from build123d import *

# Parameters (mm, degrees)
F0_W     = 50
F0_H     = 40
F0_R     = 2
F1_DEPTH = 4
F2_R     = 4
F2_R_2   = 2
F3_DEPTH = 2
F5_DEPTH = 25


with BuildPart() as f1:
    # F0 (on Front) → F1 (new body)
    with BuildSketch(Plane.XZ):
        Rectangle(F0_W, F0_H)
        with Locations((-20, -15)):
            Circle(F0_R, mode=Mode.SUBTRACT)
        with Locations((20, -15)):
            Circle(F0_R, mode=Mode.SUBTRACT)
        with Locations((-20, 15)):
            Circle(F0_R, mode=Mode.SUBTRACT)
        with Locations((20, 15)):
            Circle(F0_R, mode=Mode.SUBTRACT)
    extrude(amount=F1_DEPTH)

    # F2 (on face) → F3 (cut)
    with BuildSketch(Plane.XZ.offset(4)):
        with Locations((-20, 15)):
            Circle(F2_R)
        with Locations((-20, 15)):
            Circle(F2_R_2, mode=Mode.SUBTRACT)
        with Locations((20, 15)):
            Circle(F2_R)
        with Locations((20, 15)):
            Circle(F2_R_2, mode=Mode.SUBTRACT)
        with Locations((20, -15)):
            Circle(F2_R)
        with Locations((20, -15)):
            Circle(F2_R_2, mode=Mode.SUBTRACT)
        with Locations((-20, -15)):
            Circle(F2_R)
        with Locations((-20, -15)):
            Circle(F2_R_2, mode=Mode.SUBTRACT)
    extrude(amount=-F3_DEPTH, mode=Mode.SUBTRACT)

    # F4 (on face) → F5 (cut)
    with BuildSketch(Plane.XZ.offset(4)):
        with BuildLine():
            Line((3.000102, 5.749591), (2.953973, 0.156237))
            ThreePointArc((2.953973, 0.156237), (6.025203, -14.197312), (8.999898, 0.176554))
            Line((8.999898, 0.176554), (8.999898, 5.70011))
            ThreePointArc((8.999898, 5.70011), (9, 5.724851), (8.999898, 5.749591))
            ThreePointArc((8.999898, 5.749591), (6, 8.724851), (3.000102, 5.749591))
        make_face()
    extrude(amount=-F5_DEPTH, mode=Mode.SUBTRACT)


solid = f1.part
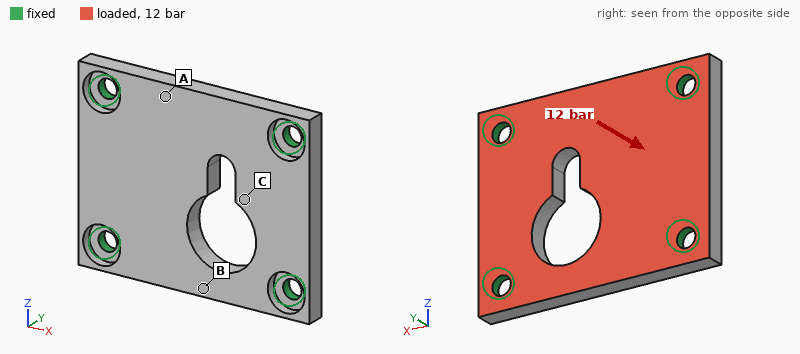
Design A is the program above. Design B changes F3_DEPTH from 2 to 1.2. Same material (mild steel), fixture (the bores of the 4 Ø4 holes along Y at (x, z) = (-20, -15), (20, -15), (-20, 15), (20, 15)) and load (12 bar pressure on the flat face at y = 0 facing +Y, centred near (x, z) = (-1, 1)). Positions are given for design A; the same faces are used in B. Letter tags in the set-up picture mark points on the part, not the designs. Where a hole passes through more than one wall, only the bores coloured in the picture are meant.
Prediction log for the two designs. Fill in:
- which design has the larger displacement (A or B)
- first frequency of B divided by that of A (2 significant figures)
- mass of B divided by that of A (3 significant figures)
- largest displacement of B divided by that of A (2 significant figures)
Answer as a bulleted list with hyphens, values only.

- A
- 1.1
- 1.02
- 0.85
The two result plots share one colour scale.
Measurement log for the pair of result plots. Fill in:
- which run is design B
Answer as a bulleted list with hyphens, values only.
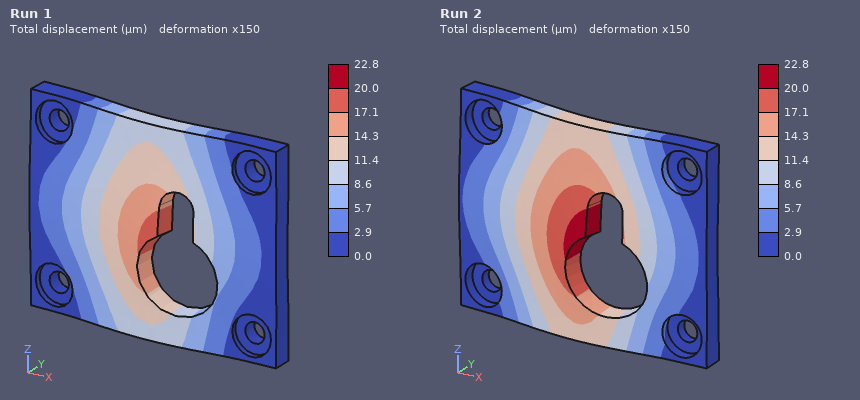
- Run 1
